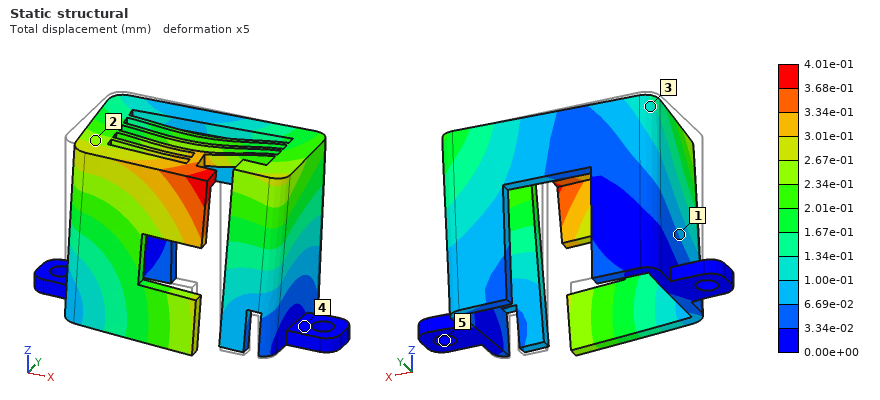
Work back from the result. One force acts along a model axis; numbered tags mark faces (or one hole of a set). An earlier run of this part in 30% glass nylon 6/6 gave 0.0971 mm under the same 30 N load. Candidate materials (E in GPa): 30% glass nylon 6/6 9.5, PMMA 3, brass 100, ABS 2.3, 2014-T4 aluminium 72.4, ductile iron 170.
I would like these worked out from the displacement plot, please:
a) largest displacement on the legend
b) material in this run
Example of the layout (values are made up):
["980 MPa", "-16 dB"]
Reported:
["4.01e-01 mm", "ABS"]
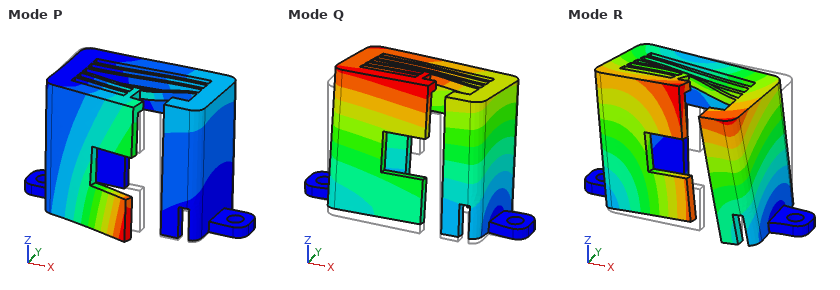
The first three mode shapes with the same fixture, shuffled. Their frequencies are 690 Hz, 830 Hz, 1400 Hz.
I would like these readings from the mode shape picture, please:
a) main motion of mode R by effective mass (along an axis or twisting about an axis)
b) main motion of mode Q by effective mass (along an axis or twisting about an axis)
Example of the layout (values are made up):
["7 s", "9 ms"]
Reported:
["along X", "along Y"]
